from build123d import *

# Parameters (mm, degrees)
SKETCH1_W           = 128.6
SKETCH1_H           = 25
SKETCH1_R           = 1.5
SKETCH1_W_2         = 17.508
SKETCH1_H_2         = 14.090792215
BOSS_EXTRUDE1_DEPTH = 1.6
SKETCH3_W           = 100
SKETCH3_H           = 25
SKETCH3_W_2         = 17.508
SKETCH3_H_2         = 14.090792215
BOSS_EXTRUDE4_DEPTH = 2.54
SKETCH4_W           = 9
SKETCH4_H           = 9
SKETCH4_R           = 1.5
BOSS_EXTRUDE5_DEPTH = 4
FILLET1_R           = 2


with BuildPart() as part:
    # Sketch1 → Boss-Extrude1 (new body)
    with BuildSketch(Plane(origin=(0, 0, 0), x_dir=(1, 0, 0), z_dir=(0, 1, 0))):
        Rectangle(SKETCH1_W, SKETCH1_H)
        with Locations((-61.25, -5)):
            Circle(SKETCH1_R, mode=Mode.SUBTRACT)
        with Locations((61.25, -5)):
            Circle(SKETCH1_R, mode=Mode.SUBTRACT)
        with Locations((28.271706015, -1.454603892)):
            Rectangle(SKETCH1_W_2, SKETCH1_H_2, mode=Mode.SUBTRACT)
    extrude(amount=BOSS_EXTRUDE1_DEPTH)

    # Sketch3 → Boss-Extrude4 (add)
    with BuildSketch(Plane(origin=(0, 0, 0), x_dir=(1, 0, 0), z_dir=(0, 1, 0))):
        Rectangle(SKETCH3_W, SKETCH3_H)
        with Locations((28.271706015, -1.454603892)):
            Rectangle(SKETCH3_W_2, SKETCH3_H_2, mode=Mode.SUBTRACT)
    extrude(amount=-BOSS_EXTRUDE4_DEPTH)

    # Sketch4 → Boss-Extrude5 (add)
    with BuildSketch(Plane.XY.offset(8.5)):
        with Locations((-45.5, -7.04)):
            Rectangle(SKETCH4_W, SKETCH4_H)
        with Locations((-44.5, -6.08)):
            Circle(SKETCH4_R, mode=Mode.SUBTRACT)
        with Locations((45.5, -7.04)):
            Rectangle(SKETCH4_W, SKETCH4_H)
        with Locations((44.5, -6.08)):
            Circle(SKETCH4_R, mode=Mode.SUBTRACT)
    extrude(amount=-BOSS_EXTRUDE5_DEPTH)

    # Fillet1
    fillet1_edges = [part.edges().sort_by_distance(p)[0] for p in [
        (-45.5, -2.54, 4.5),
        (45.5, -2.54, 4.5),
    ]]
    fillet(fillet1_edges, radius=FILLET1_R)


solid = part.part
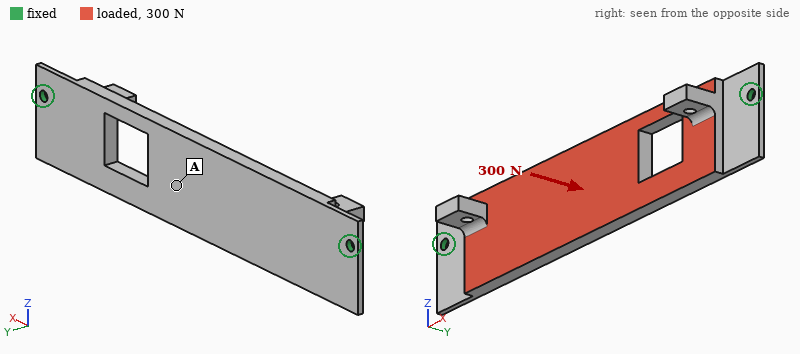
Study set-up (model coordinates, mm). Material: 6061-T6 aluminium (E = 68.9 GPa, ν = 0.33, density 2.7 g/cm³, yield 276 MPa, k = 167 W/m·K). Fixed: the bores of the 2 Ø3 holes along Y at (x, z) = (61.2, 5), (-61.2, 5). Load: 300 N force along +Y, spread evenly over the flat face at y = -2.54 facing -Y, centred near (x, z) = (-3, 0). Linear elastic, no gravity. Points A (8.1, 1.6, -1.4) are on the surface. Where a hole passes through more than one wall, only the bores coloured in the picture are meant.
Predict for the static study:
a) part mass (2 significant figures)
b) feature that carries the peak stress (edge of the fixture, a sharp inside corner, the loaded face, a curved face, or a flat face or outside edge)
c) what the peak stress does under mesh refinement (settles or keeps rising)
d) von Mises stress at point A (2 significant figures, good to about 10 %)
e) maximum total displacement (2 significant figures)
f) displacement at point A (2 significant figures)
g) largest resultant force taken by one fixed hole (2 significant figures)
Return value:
30 g
edge of the fixture
keeps rising
40 MPa
0.72 mm
0.59 mm
720 N
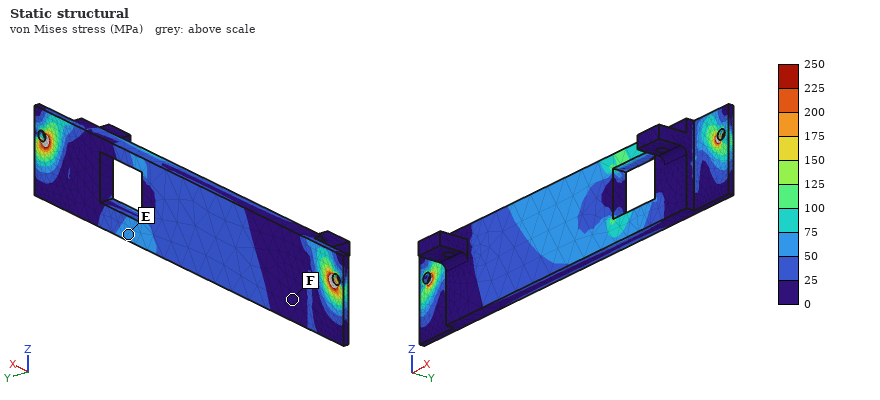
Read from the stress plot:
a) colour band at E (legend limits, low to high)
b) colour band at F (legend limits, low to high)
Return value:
50 to 75 MPa
0 to 25 MPa
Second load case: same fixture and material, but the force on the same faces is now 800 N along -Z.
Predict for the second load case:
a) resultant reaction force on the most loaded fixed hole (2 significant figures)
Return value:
500 N
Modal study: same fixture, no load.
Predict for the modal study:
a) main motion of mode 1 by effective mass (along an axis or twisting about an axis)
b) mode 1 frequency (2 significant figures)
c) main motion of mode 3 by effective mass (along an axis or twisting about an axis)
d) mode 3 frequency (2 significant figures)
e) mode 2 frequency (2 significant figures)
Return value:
along Y
780 Hz
twisting about Z
2300 Hz
1500 Hz
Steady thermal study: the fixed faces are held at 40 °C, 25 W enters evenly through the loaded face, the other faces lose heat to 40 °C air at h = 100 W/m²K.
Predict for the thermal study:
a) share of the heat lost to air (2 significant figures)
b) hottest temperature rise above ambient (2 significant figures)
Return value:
48 %
33 K
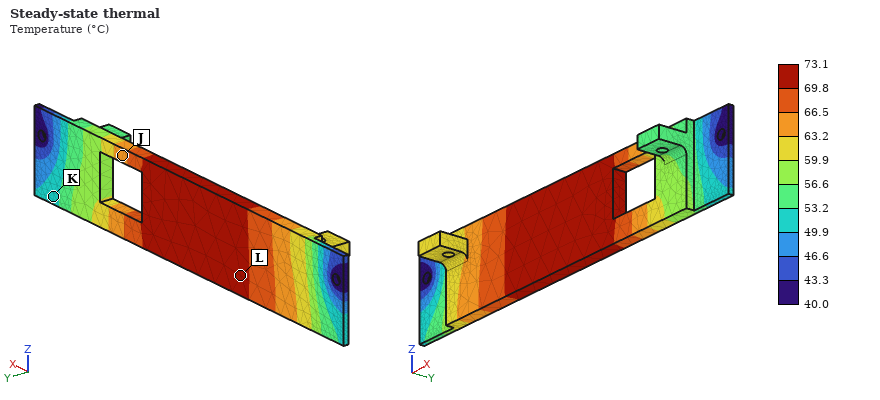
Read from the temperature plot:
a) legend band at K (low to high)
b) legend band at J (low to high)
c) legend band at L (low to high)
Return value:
49.9 to 53.2 °C
63.2 to 66.5 °C
69.8 to 73.1 °C
